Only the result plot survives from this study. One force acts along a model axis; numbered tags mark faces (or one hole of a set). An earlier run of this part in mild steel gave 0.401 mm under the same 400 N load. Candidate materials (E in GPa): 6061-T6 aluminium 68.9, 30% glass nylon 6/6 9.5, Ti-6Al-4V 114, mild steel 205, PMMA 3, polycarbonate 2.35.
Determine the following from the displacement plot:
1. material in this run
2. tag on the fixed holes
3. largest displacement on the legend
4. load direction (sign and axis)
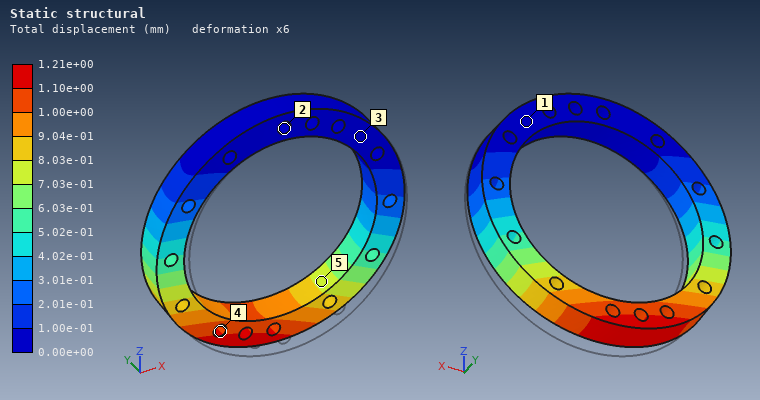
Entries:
6061-T6 aluminium
2
1.21e+00 mm
+Y
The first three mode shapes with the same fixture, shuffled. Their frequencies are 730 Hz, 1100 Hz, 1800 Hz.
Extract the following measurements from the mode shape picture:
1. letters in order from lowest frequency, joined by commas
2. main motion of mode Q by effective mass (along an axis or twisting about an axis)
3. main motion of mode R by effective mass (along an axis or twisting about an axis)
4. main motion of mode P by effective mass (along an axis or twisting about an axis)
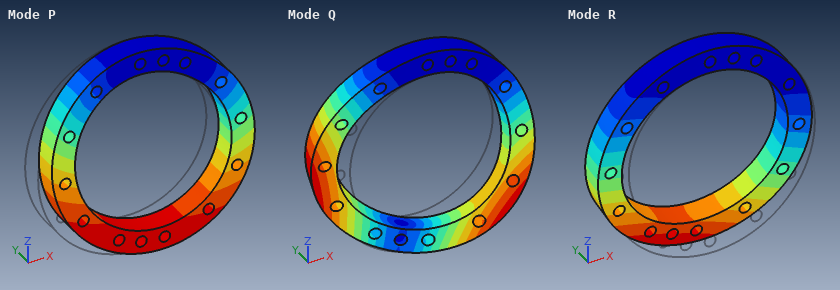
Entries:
R, P, Q
twisting about Z
along Y
along X
